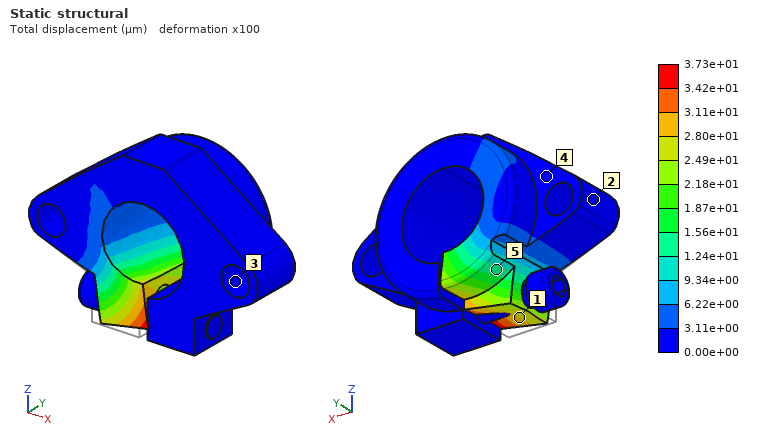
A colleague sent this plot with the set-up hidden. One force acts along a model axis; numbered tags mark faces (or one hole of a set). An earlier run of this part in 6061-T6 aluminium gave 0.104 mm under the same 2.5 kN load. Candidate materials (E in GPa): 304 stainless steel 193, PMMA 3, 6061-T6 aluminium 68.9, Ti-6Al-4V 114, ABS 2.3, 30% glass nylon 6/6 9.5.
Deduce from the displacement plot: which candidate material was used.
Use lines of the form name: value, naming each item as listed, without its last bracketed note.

which candidate material was used: 304 stainless steel
